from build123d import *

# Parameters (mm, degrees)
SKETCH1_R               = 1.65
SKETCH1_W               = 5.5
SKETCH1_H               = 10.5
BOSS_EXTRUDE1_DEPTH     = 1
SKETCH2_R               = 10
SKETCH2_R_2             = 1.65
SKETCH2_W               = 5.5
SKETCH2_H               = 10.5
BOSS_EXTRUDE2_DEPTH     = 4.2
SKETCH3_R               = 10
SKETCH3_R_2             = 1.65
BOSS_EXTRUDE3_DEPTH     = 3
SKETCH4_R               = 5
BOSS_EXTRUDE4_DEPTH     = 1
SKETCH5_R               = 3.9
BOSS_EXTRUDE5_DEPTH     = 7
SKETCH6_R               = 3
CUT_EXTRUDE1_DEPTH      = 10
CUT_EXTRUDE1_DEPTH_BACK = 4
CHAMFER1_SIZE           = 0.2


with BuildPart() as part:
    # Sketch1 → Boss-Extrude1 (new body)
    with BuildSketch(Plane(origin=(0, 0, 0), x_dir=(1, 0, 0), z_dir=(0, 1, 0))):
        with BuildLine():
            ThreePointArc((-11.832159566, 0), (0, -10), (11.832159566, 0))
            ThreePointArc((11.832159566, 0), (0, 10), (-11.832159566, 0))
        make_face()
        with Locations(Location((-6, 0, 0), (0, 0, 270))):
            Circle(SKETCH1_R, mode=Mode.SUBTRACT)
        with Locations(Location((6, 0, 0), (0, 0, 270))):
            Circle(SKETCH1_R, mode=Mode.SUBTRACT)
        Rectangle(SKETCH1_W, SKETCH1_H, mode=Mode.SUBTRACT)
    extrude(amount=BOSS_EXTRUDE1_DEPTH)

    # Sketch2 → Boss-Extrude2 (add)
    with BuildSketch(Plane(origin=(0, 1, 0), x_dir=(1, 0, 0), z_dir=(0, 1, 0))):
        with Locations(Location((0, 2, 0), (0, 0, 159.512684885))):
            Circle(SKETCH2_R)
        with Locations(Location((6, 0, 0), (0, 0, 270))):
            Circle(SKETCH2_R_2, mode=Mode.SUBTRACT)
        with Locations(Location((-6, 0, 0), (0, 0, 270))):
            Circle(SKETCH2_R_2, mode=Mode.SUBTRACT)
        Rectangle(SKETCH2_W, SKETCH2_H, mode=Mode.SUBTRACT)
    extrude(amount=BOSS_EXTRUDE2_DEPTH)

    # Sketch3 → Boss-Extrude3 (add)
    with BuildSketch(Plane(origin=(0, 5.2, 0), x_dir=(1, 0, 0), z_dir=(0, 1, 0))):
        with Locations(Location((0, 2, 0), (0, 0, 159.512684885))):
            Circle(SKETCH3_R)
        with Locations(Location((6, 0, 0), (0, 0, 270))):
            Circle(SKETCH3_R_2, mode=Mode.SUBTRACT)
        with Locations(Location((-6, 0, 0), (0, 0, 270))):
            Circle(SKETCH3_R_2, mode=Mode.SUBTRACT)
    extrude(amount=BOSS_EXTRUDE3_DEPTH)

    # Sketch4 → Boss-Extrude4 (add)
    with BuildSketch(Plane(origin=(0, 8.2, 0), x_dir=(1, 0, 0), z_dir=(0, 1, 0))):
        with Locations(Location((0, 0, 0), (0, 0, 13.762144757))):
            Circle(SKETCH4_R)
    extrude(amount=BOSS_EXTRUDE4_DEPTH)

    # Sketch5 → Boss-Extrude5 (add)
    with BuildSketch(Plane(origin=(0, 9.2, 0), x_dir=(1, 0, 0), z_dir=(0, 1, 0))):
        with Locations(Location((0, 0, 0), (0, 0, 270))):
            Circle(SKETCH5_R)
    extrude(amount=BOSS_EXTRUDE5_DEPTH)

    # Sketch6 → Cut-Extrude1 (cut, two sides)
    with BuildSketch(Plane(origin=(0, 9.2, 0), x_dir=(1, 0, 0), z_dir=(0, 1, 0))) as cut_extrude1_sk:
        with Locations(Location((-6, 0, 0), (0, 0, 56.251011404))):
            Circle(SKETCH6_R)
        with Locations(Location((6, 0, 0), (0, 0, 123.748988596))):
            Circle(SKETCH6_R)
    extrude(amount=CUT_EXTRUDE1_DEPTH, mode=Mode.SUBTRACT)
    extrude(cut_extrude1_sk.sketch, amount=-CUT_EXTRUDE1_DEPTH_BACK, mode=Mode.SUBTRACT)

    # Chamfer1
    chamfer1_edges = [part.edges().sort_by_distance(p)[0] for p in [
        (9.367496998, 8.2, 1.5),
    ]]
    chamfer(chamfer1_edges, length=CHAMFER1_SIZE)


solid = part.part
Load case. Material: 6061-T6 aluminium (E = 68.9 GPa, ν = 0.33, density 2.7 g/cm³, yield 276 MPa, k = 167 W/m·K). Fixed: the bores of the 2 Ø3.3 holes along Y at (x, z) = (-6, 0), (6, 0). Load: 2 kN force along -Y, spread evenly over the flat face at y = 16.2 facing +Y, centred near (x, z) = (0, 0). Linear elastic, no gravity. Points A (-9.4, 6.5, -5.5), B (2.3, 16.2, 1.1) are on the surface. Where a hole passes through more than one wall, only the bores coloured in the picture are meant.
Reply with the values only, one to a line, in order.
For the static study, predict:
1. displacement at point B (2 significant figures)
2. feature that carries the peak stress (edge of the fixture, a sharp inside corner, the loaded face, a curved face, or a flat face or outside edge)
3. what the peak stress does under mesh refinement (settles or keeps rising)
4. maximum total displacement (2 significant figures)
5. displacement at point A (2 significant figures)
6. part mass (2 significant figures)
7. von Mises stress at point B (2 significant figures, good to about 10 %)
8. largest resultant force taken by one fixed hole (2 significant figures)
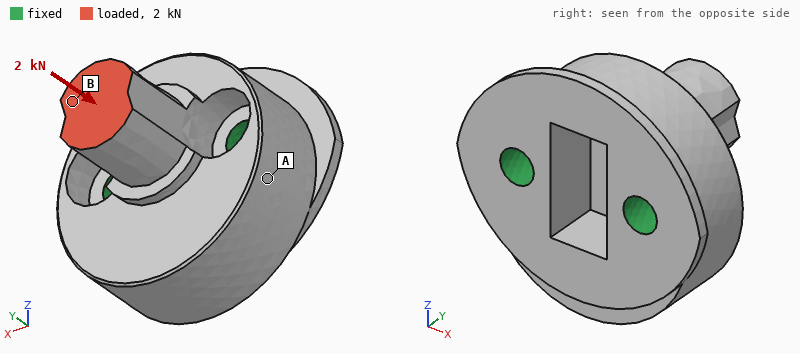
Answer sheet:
11 µm
a sharp inside corner
keeps rising
11 µm
1.7 µm
6.6 g
46 MPa
1.0 kN
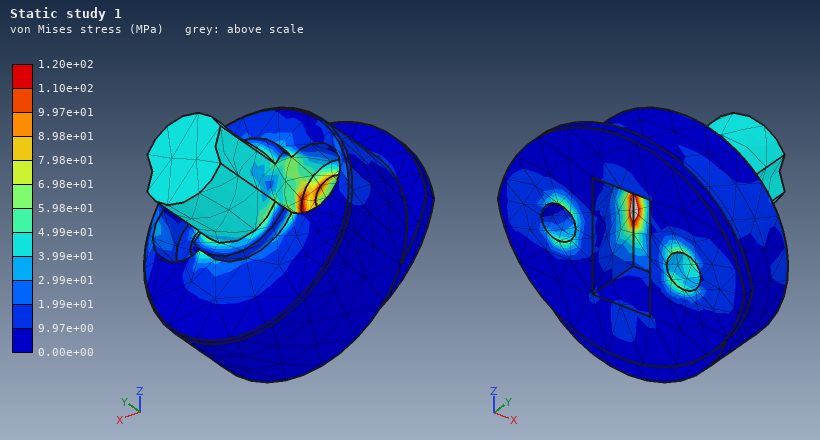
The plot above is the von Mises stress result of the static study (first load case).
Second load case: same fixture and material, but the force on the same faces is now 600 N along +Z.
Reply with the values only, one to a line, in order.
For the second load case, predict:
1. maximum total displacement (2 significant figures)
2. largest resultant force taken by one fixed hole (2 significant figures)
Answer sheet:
32 µm
300 N
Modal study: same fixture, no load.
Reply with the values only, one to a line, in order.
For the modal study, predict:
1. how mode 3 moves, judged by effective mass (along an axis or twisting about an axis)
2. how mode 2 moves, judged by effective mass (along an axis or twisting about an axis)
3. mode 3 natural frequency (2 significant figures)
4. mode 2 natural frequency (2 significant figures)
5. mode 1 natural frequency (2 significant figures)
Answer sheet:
along Y
along X
46 kHz
38 kHz
25 kHz
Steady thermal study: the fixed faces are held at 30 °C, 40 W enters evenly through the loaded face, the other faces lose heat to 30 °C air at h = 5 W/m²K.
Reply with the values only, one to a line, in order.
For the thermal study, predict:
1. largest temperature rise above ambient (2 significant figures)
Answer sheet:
63 K
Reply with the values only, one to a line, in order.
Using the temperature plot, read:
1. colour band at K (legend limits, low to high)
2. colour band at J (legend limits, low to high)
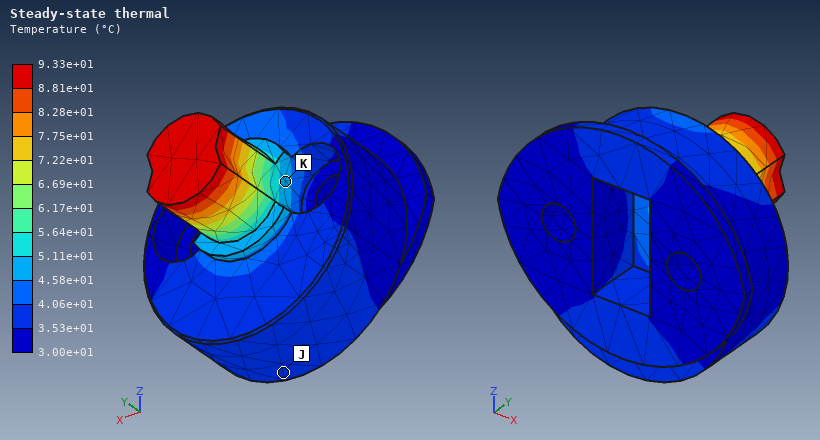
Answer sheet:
4.58e+01 to 5.11e+01 °C
3.53e+01 to 4.06e+01 °C
